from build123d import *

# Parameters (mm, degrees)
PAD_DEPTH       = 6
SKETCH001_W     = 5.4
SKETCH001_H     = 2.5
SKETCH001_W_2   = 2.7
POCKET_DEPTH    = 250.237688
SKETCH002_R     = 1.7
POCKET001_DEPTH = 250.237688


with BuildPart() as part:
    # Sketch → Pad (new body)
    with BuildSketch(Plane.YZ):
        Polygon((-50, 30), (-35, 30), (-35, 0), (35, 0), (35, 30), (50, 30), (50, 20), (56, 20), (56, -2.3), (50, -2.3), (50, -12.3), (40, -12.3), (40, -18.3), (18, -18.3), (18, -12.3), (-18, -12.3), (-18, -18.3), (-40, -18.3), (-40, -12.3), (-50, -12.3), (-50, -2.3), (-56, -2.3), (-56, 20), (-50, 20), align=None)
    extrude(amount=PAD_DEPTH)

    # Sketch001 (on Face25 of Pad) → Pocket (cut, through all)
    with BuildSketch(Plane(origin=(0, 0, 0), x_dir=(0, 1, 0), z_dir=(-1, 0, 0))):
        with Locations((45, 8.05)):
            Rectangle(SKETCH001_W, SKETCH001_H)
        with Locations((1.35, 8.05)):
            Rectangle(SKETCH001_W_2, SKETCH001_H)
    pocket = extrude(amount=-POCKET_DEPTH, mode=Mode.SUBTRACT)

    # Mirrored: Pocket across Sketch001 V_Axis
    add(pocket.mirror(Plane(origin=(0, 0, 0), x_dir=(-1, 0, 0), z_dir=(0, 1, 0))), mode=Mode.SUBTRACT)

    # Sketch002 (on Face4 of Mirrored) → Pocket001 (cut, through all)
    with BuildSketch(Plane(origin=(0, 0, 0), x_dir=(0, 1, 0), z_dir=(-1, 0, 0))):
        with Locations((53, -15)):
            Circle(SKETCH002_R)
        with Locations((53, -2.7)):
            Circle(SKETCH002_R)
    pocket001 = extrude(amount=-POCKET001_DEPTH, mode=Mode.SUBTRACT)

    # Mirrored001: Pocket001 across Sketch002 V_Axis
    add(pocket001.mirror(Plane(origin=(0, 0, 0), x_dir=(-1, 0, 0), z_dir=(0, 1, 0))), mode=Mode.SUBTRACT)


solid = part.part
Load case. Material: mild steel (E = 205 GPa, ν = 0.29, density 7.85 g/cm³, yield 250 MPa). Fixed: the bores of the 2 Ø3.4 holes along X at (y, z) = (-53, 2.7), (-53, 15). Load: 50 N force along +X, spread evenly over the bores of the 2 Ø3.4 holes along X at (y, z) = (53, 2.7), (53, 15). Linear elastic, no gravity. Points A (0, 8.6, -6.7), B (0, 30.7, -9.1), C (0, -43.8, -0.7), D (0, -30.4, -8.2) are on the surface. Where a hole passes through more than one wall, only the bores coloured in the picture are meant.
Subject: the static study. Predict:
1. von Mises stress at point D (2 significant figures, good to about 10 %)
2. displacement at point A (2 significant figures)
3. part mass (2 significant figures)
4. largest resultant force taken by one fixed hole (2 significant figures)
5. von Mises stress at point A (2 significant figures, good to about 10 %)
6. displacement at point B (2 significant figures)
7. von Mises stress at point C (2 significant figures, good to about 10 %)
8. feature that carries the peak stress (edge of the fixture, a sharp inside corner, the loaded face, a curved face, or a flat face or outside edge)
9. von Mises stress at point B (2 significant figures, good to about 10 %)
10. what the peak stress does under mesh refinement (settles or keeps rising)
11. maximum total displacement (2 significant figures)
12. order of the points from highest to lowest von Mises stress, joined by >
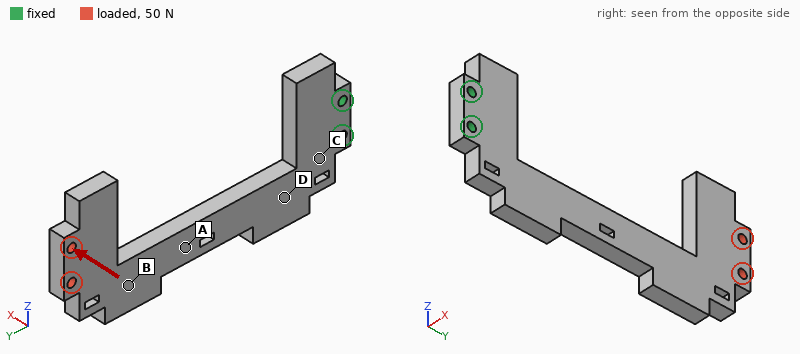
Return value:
40 MPa
0.15 mm
120 g
26 N
31 MPa
0.25 mm
48 MPa
edge of the fixture
13 MPa
keeps rising
0.42 mm
C > D > A > B
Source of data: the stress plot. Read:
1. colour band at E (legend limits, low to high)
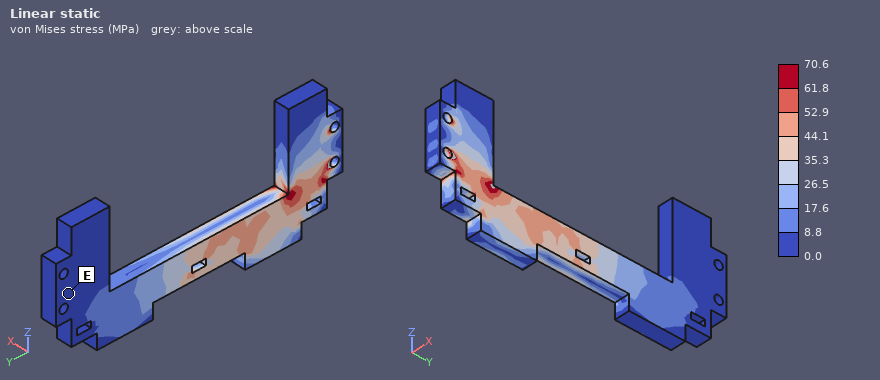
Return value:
0.0 to 8.8 MPa
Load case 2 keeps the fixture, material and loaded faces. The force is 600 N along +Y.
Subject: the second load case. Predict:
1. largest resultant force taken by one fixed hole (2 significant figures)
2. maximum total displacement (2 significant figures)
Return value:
330 N
0.21 mm
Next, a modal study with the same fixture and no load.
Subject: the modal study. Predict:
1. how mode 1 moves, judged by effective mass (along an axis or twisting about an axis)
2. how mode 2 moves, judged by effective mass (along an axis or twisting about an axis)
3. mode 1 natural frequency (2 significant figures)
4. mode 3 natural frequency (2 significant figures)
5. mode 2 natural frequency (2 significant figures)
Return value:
along X
along Z
300 Hz
1300 Hz
670 Hz
